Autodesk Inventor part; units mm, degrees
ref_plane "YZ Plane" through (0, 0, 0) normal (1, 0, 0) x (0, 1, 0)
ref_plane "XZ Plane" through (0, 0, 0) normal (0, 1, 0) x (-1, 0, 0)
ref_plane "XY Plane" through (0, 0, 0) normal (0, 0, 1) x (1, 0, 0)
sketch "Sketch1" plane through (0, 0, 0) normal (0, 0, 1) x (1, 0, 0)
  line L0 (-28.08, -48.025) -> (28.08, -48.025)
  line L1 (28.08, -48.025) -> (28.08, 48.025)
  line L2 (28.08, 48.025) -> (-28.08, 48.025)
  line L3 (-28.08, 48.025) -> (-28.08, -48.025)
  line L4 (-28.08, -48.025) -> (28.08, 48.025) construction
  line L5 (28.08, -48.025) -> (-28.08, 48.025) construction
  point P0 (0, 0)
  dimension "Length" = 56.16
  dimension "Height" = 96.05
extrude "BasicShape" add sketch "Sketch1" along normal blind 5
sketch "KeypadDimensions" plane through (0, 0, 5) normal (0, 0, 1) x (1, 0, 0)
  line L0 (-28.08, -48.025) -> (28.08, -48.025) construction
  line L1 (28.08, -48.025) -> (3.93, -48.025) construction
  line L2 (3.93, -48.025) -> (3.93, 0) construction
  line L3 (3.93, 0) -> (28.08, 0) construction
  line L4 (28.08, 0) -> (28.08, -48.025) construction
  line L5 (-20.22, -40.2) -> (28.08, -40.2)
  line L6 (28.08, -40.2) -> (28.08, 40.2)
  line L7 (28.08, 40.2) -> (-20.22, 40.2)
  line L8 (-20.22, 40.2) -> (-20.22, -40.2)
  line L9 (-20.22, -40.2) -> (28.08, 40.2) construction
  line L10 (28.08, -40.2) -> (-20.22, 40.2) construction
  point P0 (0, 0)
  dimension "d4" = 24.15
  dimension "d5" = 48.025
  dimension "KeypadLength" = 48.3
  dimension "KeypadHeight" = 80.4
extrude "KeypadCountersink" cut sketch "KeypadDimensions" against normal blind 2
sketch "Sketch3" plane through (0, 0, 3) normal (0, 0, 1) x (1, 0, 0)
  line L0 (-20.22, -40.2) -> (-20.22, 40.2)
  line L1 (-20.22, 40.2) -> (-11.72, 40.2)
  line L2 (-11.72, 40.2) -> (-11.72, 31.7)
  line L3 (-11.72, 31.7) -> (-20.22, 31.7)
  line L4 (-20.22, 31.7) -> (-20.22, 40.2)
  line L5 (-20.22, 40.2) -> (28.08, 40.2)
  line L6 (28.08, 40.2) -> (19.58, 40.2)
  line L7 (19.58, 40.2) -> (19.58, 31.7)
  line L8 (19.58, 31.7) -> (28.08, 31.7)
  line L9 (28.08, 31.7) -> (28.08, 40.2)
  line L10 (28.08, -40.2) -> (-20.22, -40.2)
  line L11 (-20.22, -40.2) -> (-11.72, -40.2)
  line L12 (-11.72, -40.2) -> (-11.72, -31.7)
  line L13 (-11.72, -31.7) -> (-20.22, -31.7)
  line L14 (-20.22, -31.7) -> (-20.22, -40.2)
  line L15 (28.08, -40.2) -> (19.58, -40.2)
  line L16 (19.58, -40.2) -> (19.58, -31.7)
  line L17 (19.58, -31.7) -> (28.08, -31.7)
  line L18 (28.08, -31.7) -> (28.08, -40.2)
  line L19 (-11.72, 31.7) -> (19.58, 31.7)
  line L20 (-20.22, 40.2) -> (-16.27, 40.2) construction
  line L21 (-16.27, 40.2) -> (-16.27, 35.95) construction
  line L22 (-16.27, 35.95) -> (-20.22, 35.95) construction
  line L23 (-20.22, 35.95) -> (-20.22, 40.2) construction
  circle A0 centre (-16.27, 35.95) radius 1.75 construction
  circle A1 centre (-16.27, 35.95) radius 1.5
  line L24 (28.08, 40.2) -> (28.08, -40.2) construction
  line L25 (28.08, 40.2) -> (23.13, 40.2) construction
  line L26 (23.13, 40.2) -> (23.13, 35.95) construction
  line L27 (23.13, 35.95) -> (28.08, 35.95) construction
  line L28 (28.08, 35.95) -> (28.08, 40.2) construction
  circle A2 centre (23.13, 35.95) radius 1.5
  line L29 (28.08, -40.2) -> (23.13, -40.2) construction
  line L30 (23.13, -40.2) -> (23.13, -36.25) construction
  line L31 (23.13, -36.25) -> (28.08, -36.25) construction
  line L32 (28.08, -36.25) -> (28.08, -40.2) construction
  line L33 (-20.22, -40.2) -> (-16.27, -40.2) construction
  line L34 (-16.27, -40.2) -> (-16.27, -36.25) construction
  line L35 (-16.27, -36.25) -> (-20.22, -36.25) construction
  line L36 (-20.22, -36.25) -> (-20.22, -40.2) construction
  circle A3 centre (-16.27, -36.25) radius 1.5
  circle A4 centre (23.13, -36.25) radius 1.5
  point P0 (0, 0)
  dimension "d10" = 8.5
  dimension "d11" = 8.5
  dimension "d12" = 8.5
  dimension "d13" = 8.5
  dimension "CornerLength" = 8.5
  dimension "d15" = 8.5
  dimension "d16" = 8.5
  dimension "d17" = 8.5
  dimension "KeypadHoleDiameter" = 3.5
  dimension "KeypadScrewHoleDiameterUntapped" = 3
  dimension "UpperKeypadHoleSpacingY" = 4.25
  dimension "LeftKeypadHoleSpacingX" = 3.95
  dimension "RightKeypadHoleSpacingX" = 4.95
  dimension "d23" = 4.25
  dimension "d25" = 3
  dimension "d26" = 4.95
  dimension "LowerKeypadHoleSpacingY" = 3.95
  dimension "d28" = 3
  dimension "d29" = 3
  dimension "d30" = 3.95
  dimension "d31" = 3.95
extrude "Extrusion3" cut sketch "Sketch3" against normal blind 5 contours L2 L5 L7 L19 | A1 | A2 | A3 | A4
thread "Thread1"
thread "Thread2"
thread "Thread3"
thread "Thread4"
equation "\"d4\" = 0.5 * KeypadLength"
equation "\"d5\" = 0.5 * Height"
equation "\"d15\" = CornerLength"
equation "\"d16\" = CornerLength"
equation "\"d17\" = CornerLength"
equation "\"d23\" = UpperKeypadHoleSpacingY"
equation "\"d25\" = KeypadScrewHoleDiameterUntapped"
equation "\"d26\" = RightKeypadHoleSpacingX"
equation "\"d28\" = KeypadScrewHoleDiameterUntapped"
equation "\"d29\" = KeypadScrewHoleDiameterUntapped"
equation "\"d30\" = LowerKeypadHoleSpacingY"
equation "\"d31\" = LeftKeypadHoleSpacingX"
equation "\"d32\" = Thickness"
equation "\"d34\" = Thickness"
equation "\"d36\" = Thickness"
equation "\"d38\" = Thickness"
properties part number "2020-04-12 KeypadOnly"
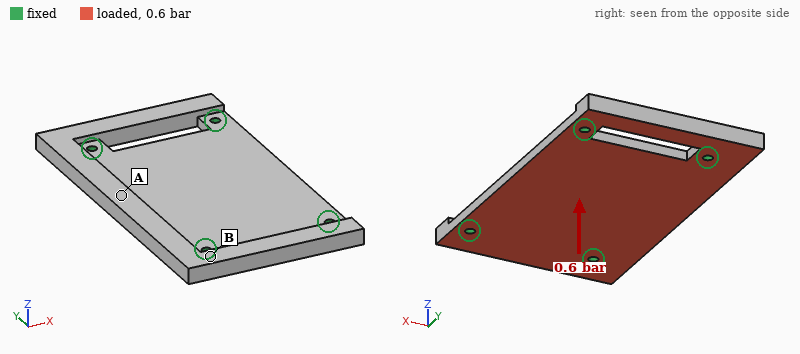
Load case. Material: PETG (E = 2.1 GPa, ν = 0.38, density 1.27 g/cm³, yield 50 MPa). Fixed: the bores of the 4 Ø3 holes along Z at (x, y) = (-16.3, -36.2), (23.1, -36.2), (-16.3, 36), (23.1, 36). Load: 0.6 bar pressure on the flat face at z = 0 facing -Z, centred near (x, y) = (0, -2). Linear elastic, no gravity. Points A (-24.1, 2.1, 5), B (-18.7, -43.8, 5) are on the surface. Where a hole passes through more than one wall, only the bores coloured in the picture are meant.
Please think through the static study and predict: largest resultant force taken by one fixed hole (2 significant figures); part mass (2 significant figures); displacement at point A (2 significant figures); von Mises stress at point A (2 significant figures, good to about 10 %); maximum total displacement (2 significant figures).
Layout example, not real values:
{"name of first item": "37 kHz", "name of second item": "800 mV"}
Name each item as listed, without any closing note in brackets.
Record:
{"largest resultant force taken by one fixed hole": "97 N", "part mass": "23 g", "displacement at point A": "0.65 mm", "von Mises stress at point A": "10.0 MPa", "maximum total displacement": "1.2 mm"}
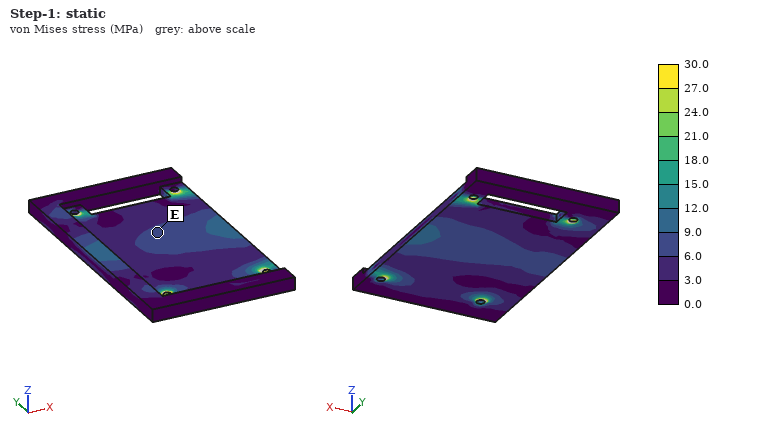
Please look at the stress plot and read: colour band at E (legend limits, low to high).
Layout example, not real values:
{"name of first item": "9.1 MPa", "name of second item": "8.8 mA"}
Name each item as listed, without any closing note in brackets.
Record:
{"colour band at E": "6.0 to 9.0 MPa"}
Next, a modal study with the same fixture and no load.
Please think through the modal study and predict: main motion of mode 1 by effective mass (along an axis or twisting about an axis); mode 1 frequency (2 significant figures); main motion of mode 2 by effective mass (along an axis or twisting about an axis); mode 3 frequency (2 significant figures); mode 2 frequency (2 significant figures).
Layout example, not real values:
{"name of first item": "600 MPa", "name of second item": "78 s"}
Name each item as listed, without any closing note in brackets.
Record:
{"main motion of mode 1 by effective mass": "along Z", "mode 1 frequency": "700 Hz", "main motion of mode 2 by effective mass": "twisting about Y", "mode 3 frequency": "1700 Hz", "mode 2 frequency": "1000 Hz"}
